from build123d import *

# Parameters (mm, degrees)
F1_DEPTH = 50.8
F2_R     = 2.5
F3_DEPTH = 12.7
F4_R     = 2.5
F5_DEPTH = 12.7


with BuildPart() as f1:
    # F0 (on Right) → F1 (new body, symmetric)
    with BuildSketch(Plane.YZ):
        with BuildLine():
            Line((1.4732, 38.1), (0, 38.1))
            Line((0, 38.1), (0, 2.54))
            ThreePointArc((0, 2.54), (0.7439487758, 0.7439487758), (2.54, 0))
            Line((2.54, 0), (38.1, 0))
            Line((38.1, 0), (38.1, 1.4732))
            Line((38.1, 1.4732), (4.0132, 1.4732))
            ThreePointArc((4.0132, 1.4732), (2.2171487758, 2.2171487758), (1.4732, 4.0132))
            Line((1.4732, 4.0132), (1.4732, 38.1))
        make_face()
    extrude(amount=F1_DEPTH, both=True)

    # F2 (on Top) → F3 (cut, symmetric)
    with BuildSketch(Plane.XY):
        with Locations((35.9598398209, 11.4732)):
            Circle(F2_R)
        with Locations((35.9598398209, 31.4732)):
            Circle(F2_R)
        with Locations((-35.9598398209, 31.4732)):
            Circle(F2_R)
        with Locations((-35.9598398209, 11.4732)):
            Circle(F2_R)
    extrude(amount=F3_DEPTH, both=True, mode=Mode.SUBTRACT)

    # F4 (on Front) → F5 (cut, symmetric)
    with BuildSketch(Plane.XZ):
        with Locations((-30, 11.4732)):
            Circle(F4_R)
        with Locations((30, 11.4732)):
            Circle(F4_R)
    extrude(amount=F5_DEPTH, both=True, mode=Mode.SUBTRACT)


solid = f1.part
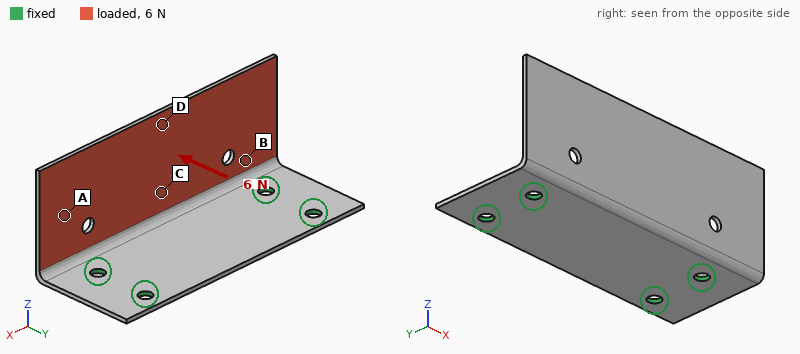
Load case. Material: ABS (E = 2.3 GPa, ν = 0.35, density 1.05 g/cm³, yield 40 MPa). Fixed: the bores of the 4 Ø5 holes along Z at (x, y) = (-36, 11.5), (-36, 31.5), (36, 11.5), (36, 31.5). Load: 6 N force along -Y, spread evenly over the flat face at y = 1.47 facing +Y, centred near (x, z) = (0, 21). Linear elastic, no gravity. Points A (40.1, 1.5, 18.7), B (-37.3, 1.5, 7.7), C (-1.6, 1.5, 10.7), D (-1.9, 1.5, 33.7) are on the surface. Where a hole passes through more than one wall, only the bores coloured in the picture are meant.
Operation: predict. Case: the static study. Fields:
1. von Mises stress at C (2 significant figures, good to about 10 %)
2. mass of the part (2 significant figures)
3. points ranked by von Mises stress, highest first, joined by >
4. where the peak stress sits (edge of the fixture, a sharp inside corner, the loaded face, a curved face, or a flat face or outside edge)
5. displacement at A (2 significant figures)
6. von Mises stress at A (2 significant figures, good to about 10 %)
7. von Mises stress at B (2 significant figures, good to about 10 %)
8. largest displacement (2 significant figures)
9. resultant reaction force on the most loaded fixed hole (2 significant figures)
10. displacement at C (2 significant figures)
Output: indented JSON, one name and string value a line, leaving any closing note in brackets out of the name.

{
  "von Mises stress at C": "1.6 MPa",
  "mass of the part": "12 g",
  "points ranked by von Mises stress, highest first, joined by >": "B > C > A > D",
  "where the peak stress sits": "a flat face or outside edge",
  "displacement at A": "0.51 mm",
  "von Mises stress at A": "0.87 MPa",
  "von Mises stress at B": "2.0 MPa",
  "largest displacement": "1.3 mm",
  "resultant reaction force on the most loaded fixed hole": "2.4 N",
  "displacement at C": "0.27 mm"
}
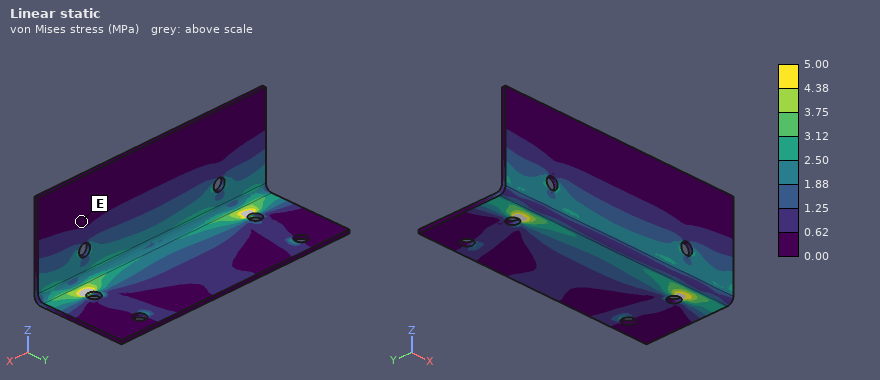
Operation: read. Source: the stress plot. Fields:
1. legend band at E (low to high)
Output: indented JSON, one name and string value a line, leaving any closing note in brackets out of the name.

{
  "legend band at E": "0.00 to 0.62 MPa"
}
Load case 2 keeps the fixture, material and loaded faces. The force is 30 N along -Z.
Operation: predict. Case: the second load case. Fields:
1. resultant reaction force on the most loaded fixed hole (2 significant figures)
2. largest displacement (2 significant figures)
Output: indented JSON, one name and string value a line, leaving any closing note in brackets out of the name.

{
  "resultant reaction force on the most loaded fixed hole": "17 N",
  "largest displacement": "0.90 mm"
}
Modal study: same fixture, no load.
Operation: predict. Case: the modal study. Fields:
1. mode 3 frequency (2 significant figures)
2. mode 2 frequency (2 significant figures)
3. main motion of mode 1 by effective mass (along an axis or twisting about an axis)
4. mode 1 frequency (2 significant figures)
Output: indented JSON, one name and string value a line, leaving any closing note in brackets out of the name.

{
  "mode 3 frequency": "500 Hz",
  "mode 2 frequency": "280 Hz",
  "main motion of mode 1 by effective mass": "along Y",
  "mode 1 frequency": "180 Hz"
}
